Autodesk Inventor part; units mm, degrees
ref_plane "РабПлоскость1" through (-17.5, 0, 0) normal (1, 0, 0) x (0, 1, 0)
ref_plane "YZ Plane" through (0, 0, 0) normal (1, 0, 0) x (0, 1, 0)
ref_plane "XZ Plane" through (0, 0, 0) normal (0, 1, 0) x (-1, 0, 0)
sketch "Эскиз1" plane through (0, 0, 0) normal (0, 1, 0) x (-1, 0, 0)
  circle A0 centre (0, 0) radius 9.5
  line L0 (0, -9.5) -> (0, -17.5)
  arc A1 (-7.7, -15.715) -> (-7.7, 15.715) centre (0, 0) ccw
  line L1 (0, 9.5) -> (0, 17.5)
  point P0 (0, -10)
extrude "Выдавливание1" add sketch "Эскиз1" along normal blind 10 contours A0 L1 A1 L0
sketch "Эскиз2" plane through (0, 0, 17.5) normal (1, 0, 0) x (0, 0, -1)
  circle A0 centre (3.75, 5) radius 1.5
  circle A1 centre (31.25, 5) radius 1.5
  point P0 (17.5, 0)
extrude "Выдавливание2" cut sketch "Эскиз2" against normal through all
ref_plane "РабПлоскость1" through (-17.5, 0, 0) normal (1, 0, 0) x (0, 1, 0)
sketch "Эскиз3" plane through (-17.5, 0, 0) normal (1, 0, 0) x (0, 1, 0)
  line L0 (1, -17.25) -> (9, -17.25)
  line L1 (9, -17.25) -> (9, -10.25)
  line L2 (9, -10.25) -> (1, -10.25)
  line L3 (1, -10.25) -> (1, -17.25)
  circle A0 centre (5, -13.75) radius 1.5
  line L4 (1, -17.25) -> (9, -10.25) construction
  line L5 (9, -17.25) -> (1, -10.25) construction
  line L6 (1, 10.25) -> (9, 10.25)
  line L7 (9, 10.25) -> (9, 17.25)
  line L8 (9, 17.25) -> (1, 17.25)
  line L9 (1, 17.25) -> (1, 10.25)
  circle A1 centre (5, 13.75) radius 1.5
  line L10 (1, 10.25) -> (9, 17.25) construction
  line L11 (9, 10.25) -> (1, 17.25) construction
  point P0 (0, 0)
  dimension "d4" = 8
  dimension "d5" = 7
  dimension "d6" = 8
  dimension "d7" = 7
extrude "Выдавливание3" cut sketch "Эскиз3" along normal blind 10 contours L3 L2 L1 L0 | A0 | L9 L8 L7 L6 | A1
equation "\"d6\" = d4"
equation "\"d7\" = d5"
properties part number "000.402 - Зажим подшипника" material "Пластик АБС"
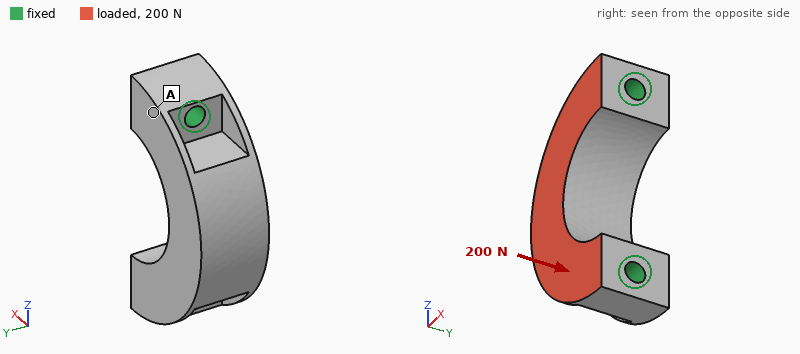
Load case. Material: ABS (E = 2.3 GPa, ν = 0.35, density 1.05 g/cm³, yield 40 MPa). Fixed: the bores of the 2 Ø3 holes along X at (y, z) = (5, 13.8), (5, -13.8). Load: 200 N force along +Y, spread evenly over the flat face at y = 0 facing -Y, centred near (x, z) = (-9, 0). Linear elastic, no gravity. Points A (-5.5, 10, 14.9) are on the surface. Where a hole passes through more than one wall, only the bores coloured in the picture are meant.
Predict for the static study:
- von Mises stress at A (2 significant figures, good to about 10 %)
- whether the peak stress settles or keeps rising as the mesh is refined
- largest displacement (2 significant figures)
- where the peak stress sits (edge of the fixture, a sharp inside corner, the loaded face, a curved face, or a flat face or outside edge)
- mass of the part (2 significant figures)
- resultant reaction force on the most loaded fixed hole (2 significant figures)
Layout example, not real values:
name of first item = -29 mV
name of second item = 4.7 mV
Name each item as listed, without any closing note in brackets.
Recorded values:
von Mises stress at A = 2.4 MPa
whether the peak stress settles or keeps rising as the mesh is refined = keeps rising
largest displacement = 95 µm
where the peak stress sits = edge of the fixture
mass of the part = 3.1 g
resultant reaction force on the most loaded fixed hole = 100 N
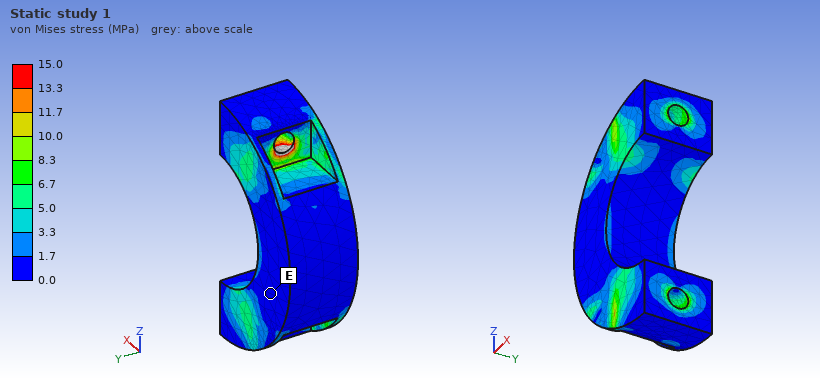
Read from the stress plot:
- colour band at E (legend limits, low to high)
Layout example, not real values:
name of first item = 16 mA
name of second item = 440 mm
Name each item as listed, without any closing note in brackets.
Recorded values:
colour band at E = 0.0 to 1.7 MPa
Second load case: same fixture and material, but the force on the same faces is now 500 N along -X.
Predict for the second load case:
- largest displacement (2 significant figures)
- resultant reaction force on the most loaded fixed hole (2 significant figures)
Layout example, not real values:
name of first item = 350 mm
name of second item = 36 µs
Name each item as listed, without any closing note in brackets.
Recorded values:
largest displacement = 0.18 mm
resultant reaction force on the most loaded fixed hole = 260 N
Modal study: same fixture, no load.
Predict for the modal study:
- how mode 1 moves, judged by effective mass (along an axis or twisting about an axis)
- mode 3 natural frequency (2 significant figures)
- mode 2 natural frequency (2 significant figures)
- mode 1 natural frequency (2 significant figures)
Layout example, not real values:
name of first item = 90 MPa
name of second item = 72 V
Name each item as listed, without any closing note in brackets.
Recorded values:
how mode 1 moves, judged by effective mass = along Y
mode 3 natural frequency = 12 kHz
mode 2 natural frequency = 12 kHz
mode 1 natural frequency = 4900 Hz
